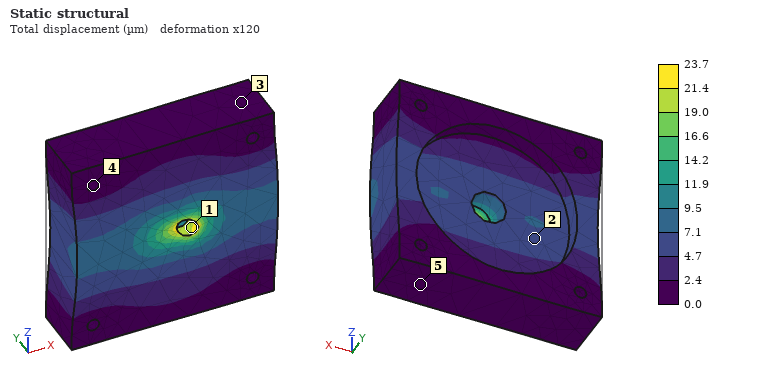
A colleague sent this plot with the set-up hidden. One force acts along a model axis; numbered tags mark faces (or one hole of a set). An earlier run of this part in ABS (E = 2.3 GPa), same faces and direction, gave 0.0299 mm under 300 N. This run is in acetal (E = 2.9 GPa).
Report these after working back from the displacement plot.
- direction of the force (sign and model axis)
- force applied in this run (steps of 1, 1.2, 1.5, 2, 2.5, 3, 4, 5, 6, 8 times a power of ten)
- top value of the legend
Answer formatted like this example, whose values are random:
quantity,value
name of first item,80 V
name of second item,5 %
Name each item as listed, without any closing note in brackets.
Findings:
quantity,value
direction of the force,+X
force applied in this run,300 N
top value of the legend,23.7 µm
